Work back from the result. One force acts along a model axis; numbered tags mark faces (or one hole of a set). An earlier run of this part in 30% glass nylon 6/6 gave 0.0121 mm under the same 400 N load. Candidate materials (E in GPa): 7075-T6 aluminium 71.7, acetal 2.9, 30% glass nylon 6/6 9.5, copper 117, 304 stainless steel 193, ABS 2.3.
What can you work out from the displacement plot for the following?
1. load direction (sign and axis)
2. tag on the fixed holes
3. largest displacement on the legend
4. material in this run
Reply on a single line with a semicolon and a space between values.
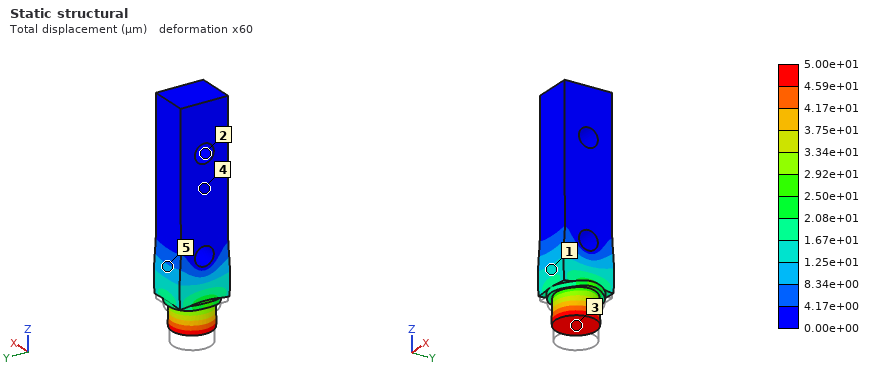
+Z; 2; 5.00e+01 µm; ABS
